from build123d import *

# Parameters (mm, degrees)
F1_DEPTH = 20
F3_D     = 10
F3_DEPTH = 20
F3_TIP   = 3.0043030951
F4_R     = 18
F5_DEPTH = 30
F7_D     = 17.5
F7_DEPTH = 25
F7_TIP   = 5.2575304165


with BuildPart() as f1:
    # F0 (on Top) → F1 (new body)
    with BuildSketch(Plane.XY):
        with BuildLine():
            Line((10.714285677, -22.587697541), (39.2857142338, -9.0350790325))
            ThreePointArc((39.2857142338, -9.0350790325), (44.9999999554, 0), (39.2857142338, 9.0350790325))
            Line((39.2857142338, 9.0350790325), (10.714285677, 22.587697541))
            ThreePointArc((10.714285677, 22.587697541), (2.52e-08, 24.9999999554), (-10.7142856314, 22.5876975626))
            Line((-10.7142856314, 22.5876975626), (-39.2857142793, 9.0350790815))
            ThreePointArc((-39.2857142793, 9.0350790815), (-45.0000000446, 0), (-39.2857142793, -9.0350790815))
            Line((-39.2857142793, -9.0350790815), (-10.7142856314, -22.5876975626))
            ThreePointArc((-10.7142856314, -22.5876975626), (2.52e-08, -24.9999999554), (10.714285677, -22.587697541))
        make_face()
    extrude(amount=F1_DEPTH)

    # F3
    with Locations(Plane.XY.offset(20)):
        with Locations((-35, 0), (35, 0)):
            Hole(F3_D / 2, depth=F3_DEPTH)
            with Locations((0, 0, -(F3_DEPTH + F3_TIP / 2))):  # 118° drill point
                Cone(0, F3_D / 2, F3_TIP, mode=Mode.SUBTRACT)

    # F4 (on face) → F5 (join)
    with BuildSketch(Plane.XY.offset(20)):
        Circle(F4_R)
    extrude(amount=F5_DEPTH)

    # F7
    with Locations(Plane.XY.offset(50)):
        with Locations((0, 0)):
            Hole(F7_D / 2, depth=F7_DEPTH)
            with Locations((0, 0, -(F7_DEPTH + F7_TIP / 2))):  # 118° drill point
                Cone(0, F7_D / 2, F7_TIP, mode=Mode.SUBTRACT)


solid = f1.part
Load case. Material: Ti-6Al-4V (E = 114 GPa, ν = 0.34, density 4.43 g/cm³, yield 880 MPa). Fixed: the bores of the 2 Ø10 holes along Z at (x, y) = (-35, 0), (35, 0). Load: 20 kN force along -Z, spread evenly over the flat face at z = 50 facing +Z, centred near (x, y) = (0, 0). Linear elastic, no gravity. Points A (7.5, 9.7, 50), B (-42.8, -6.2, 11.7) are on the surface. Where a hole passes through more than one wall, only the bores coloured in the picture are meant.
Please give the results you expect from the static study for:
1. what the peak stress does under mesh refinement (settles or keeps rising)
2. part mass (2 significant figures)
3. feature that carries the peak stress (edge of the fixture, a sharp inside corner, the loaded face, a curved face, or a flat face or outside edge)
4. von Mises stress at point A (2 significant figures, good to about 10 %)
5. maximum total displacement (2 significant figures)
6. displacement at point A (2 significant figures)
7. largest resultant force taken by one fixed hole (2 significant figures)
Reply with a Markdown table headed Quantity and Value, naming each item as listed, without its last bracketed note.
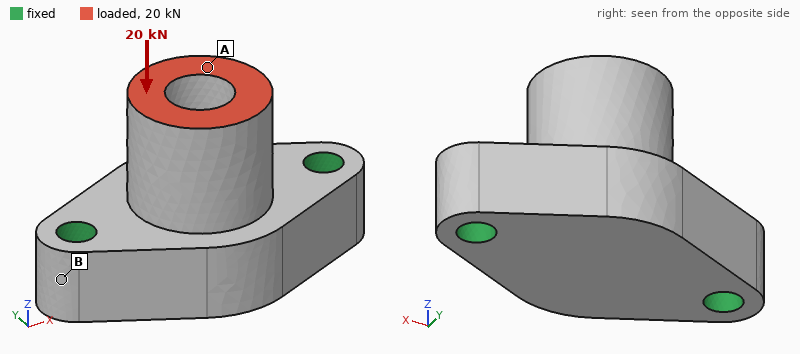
| Quantity | Value |
|---|---|
| what the peak stress does under mesh refinement | keeps rising |
| part mass | 360 g |
| feature that carries the peak stress | edge of the fixture |
| von Mises stress at point A | 26 MPa |
| maximum total displacement | 22 µm |
| displacement at point A | 21 µm |
| largest resultant force taken by one fixed hole | 10 kN |
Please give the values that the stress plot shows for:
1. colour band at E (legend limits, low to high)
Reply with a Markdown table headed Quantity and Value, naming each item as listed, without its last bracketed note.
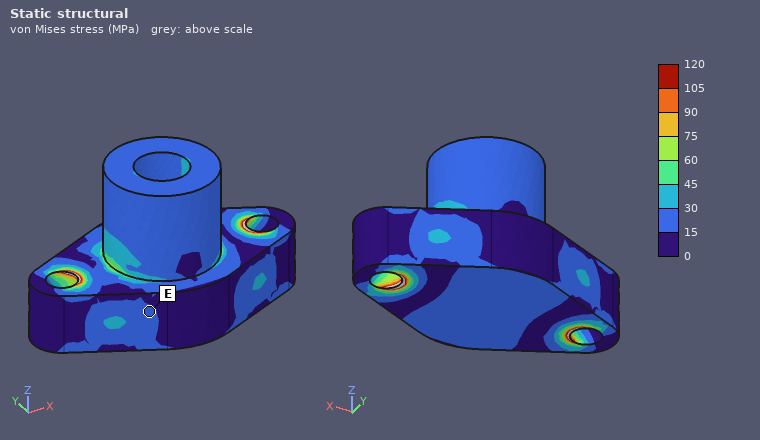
| Quantity | Value |
|---|---|
| colour band at E | 15 to 30 MPa |
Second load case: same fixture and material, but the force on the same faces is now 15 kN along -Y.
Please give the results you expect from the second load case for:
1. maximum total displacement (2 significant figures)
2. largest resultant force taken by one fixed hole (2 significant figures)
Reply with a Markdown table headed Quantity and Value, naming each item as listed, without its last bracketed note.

| Quantity | Value |
|---|---|
| maximum total displacement | 0.18 mm |
| largest resultant force taken by one fixed hole | 7.5 kN |
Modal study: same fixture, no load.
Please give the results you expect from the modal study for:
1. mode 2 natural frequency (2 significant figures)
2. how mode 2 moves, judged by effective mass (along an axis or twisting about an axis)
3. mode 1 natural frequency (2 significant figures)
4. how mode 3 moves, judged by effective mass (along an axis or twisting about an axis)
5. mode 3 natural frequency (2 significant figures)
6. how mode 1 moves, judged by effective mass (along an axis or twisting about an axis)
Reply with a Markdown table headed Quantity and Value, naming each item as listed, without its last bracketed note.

| Quantity | Value |
|---|---|
| mode 2 natural frequency | 11 kHz |
| how mode 2 moves, judged by effective mass | along Z |
| mode 1 natural frequency | 6200 Hz |
| how mode 3 moves, judged by effective mass | along X |
| mode 3 natural frequency | 12 kHz |
| how mode 1 moves, judged by effective mass | along Y |
